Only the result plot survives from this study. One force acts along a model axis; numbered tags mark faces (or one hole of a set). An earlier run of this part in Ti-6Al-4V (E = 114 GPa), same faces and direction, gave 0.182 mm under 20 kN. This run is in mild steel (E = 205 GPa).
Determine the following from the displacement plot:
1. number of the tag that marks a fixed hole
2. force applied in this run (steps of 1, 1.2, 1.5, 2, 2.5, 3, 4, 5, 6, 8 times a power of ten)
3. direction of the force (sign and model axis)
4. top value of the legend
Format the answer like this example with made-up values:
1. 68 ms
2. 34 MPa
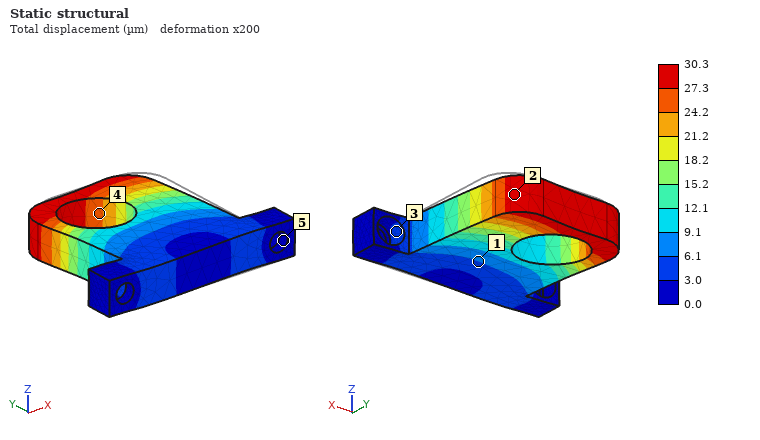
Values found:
1. 5
2. 6 kN
3. -X
4. 30.3 µm
